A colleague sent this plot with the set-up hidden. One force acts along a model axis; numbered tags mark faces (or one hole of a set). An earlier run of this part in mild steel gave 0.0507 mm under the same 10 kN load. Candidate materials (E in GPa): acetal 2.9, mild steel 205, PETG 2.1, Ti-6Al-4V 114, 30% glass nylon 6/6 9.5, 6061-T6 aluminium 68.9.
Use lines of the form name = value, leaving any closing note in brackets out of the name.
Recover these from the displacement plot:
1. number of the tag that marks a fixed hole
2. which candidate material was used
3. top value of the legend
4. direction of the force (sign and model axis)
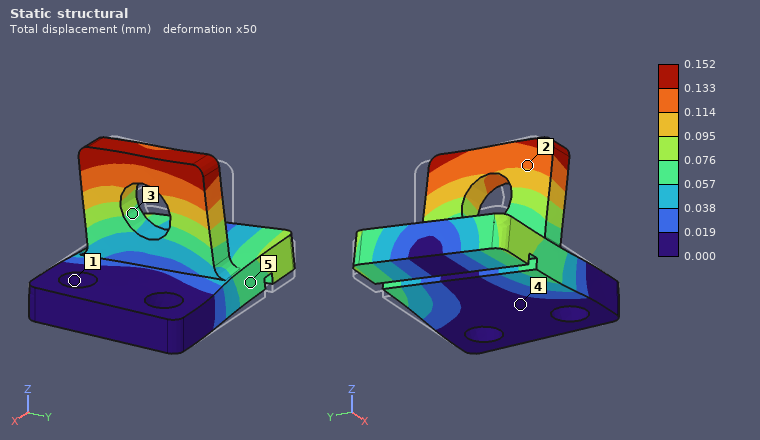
number of the tag that marks a fixed hole = 1
which candidate material was used = 6061-T6 aluminium
top value of the legend = 0.152 mm
direction of the force = -Y
